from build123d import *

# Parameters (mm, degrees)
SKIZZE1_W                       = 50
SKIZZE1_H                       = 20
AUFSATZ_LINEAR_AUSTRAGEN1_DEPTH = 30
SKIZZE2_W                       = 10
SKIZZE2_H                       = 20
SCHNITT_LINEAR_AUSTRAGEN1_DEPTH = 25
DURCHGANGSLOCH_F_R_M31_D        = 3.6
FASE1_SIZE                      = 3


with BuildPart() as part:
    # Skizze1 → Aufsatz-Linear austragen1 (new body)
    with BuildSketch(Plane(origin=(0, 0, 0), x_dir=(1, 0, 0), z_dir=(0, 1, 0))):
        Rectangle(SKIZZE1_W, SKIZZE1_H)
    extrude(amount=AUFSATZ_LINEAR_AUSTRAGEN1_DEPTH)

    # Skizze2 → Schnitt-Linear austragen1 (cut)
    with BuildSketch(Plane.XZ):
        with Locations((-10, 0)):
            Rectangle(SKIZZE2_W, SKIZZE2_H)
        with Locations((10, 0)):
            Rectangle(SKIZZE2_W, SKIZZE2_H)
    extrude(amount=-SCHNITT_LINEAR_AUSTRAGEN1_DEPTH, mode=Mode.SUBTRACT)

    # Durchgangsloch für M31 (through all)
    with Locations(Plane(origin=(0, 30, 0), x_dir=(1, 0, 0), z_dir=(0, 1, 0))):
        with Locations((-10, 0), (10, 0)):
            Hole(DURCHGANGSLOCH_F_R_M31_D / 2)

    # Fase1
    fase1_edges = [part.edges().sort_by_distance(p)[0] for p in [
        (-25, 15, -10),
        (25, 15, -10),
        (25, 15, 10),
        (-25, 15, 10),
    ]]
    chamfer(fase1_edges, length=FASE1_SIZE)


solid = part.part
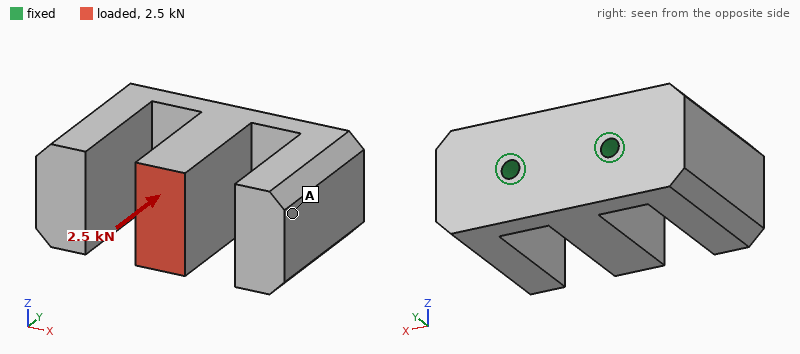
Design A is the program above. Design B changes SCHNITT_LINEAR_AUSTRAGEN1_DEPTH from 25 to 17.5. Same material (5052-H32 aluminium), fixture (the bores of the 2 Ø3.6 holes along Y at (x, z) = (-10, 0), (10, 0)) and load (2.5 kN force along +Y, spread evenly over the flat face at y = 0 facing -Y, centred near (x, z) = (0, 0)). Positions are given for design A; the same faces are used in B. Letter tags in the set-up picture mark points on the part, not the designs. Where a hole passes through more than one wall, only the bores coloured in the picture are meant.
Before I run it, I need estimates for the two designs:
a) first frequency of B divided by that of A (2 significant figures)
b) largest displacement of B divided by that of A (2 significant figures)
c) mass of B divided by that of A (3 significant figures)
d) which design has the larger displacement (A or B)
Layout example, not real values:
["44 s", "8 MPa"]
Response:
["3.3", "0.40", "1.15", "A"]
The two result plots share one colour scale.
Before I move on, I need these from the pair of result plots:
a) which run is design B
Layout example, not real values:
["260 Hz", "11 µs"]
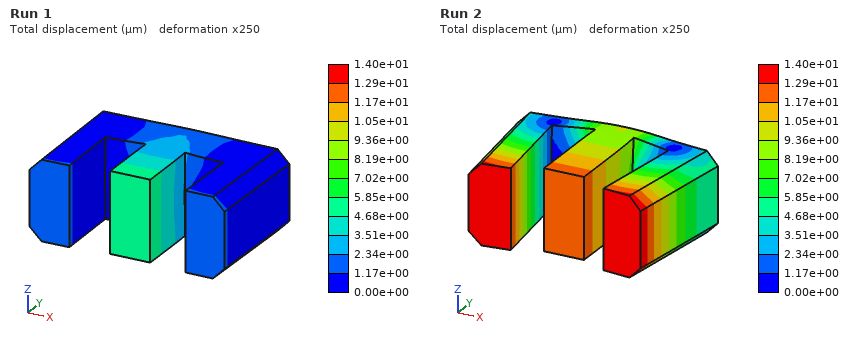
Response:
["Run 1"]
